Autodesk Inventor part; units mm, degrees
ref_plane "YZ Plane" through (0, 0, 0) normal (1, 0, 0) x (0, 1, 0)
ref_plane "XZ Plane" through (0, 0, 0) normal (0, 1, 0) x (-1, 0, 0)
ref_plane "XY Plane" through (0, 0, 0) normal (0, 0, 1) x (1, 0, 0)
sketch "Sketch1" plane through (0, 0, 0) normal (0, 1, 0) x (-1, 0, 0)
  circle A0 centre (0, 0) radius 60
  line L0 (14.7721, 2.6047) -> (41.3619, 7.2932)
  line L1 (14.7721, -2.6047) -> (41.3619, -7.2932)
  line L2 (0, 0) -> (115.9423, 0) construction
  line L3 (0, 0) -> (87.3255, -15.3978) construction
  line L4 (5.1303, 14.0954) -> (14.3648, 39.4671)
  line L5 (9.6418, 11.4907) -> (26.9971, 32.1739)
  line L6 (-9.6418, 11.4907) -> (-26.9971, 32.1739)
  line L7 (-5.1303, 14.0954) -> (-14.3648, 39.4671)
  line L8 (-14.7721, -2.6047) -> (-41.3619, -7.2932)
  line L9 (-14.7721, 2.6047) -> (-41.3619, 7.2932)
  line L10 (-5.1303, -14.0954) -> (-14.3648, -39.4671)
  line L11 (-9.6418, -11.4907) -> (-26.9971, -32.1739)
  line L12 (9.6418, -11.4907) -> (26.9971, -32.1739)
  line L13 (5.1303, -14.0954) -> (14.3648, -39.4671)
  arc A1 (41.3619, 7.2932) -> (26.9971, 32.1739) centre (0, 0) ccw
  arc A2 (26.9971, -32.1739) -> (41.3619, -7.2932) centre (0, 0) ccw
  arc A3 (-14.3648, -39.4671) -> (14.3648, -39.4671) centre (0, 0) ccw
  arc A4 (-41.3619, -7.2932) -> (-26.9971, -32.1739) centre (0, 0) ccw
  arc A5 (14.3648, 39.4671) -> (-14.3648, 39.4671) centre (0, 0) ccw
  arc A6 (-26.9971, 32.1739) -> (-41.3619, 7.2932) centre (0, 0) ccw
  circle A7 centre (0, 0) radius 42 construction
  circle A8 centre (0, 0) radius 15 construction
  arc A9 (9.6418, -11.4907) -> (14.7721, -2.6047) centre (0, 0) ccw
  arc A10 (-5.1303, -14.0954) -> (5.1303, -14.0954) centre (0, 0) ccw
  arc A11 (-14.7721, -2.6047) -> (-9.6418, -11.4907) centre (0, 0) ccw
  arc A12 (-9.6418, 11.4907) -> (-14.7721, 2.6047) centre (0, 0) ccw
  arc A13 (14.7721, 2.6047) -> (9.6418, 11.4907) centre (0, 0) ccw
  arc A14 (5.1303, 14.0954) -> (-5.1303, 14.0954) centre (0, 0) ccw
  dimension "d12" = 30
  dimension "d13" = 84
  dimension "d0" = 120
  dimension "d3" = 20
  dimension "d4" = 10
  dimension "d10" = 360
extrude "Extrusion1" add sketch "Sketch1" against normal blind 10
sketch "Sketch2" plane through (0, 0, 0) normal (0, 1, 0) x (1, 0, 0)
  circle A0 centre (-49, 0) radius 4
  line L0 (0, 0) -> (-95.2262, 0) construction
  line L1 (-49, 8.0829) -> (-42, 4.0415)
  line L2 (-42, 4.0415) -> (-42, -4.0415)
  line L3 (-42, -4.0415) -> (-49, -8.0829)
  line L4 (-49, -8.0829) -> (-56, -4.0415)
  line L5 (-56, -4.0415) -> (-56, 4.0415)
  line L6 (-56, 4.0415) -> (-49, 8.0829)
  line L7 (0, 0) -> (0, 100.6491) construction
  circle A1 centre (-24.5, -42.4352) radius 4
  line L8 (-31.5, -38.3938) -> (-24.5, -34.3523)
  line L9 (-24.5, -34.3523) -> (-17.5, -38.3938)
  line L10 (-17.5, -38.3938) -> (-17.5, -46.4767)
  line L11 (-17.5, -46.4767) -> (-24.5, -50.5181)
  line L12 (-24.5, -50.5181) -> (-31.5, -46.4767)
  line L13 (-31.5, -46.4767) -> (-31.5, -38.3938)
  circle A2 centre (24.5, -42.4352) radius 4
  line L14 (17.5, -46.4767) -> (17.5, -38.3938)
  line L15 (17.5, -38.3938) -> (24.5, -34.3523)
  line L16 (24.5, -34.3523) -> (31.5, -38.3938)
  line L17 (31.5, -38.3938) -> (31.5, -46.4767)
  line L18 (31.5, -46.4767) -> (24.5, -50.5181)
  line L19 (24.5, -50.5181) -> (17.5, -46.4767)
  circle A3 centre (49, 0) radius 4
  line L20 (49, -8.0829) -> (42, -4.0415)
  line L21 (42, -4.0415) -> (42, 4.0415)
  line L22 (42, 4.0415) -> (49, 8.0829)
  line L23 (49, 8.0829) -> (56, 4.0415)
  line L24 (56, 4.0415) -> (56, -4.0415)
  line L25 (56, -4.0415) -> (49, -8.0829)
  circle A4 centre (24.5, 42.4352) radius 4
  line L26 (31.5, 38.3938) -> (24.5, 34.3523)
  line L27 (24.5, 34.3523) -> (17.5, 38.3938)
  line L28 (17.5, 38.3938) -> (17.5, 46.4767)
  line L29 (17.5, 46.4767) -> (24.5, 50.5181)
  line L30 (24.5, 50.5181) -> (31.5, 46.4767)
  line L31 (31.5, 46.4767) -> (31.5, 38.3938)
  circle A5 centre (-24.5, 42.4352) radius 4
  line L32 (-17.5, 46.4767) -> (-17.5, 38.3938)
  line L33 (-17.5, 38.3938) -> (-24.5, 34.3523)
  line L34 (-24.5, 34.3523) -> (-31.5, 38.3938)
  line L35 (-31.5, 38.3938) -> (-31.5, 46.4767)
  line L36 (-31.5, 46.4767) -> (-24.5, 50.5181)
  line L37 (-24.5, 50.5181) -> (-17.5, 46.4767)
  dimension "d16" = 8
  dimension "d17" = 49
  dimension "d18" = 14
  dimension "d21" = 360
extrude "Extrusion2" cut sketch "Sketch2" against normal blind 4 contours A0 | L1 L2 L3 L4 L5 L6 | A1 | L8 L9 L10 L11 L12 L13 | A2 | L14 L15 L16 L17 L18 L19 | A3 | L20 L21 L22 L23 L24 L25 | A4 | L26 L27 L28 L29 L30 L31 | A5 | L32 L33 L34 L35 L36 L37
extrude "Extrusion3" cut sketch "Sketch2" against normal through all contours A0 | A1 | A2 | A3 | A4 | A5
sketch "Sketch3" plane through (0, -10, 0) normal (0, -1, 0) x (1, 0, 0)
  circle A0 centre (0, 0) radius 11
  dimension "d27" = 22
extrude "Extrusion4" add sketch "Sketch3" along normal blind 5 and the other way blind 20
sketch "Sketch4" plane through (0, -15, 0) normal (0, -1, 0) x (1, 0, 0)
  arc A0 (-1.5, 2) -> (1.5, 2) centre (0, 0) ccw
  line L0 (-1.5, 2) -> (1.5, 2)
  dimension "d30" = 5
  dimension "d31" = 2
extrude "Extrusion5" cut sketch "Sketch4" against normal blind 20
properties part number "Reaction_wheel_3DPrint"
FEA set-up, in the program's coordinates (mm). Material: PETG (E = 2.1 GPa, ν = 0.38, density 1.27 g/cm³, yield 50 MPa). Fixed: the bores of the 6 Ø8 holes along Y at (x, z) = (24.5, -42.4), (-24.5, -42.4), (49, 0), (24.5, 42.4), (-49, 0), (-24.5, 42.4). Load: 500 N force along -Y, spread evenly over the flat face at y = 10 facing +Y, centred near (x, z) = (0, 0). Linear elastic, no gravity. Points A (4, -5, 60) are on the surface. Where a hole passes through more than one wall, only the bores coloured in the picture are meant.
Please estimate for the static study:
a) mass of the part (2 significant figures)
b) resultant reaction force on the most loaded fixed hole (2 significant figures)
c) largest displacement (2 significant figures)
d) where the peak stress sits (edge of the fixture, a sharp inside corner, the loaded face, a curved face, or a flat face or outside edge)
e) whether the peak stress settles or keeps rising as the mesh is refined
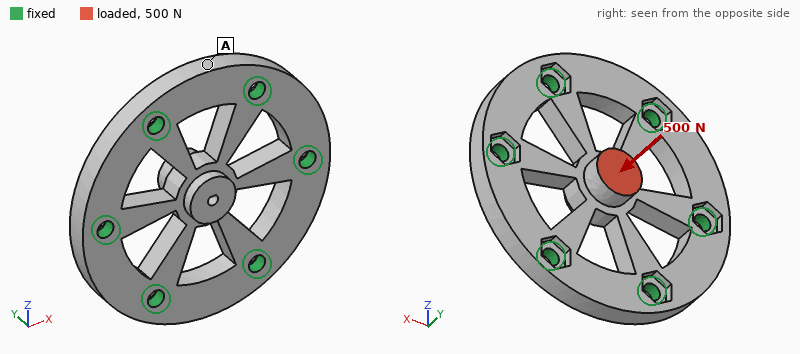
100 g
120 N
0.31 mm
edge of the fixture
keeps rising
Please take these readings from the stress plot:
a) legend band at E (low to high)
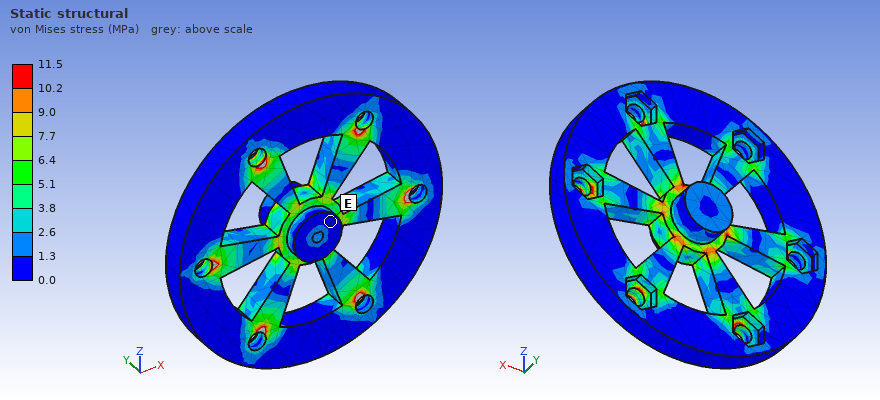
0.0 to 1.3 MPa
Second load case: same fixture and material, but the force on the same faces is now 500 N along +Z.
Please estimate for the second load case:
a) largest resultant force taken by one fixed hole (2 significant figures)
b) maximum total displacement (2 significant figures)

150 N
0.22 mm
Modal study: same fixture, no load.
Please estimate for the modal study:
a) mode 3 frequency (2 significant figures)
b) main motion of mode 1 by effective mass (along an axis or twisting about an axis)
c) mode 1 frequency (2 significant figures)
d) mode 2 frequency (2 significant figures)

2900 Hz
along Y
1400 Hz
2900 Hz
